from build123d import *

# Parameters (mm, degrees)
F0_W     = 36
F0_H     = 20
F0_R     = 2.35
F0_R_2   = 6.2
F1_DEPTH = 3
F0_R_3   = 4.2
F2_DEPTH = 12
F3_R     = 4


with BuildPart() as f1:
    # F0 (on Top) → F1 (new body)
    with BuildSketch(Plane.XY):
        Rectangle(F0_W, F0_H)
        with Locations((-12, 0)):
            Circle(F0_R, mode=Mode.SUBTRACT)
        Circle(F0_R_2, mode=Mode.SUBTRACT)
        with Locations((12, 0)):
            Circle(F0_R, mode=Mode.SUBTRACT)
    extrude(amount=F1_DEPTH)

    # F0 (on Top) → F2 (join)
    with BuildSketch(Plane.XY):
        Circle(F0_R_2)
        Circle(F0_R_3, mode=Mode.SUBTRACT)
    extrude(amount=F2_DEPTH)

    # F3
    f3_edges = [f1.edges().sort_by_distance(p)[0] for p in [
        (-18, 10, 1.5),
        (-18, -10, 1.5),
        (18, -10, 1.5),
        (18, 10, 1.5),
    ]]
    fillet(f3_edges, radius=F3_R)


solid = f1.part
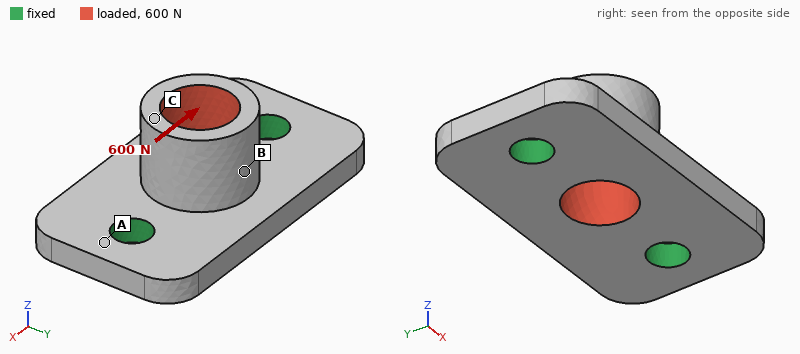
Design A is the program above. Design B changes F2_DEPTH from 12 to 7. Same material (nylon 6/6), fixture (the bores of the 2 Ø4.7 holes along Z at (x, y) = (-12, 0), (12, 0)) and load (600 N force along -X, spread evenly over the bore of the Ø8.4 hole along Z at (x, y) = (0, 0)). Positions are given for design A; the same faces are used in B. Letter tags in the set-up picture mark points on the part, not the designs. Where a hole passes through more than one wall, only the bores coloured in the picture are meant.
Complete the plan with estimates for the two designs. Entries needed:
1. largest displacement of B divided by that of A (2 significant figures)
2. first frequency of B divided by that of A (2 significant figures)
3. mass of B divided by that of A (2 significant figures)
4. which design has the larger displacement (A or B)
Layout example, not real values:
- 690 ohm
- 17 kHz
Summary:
- 0.36
- 1.3
- 0.87
- A
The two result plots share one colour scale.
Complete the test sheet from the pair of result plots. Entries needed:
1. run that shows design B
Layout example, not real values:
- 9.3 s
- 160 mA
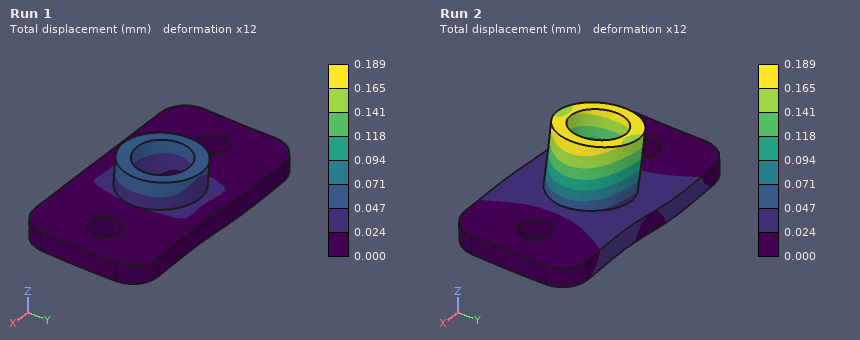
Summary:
- Run 1
